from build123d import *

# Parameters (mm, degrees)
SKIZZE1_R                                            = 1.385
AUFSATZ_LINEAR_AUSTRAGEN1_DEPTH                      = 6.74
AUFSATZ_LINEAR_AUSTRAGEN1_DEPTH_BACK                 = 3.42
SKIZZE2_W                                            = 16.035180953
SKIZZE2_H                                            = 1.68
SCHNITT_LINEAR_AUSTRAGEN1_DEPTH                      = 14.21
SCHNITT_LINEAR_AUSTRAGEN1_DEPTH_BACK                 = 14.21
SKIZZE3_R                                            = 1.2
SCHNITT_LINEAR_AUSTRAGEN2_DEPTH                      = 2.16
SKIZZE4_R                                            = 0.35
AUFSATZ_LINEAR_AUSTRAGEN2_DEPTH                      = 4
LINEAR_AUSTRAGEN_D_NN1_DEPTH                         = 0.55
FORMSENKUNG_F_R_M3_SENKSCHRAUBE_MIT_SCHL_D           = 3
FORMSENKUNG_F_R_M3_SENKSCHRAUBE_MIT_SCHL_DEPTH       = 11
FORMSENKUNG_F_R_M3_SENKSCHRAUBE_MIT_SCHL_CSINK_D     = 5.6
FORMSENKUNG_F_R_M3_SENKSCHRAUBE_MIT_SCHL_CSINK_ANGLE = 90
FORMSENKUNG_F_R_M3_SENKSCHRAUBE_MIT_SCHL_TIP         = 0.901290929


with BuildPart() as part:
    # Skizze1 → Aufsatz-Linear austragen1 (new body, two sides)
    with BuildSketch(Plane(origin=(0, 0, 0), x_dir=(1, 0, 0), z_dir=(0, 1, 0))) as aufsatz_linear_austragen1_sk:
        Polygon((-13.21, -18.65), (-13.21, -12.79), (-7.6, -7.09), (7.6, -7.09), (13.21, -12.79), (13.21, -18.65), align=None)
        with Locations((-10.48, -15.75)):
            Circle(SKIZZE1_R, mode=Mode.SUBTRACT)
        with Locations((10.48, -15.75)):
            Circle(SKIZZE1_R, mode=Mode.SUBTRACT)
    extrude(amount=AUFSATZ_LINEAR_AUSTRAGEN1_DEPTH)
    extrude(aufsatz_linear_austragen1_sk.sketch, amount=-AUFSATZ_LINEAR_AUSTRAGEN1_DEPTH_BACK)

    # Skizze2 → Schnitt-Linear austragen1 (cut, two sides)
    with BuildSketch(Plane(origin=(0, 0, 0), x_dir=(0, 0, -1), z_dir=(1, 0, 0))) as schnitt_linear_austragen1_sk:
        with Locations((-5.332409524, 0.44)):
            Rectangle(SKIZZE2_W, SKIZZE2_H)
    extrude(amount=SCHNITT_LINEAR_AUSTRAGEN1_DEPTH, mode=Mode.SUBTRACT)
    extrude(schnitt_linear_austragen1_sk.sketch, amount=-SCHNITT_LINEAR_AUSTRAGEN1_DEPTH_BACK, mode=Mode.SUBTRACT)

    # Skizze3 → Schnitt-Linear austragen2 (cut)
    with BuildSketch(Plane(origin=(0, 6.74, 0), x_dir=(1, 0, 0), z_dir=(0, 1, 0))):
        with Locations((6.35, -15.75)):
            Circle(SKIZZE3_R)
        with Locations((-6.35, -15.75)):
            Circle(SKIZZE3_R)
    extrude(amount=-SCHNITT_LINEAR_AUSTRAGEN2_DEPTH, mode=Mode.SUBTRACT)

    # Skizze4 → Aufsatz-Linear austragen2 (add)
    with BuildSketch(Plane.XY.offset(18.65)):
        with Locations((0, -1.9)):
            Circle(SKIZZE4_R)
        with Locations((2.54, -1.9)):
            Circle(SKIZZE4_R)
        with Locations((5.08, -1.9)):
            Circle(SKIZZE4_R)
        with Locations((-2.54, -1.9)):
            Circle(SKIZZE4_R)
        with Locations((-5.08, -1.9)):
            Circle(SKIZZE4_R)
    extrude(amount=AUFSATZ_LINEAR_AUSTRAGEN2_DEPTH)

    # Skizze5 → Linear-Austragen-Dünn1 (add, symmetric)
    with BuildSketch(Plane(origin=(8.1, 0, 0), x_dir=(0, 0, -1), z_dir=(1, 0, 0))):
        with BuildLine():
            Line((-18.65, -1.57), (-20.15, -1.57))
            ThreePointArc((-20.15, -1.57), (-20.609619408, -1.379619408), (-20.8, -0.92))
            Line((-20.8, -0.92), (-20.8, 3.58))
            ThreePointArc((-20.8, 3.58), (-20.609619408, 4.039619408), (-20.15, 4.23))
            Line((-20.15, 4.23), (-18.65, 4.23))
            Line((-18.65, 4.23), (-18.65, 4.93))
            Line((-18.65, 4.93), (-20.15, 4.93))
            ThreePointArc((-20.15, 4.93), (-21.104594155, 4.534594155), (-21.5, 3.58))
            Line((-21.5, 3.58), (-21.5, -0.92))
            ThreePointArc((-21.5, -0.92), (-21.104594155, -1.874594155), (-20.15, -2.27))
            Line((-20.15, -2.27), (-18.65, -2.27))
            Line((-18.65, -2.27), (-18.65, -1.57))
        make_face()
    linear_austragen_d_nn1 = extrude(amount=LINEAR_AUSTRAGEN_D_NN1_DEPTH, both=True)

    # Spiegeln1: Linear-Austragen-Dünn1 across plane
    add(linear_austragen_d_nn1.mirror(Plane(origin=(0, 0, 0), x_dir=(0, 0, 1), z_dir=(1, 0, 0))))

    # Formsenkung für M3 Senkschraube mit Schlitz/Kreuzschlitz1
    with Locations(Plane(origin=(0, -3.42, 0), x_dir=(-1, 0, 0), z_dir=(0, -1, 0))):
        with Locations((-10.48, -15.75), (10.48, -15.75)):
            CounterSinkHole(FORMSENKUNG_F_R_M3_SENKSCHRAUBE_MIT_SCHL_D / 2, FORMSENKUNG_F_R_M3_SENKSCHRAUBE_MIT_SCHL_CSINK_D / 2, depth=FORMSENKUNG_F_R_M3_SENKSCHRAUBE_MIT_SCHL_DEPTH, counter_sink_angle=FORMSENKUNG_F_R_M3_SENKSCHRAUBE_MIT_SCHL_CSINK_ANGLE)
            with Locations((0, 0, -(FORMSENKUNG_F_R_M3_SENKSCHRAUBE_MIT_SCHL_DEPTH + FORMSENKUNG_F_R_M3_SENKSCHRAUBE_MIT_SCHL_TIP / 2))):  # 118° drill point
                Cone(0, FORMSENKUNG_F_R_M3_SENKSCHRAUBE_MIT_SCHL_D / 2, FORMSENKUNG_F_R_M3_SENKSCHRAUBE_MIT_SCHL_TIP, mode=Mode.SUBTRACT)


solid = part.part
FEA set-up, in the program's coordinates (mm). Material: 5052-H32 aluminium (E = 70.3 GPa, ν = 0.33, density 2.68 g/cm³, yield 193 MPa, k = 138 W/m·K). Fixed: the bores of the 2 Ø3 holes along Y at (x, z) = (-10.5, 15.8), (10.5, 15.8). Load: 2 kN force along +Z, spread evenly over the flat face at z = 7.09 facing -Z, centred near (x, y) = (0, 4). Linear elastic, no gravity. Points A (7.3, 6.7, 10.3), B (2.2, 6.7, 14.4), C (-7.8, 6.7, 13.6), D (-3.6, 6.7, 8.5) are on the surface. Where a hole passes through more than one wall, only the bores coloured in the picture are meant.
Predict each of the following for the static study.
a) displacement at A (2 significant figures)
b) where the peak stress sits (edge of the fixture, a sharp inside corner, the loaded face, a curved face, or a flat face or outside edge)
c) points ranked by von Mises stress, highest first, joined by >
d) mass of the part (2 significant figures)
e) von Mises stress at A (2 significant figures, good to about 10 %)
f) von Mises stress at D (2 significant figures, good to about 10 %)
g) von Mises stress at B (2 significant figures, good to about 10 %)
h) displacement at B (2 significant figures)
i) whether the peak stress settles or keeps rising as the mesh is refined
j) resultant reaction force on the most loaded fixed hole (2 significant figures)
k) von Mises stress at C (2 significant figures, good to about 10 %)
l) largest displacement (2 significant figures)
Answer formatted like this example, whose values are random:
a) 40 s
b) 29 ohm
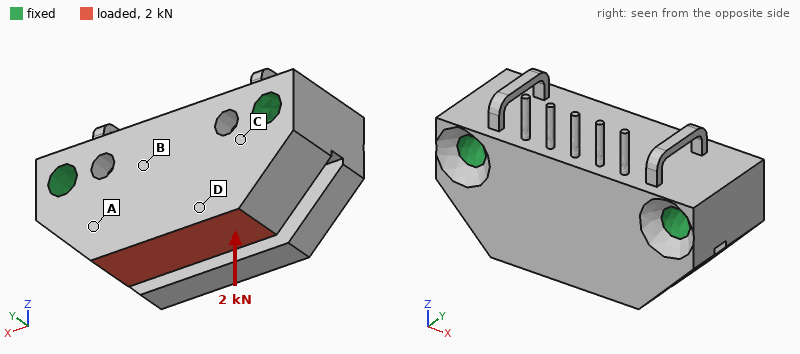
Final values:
a) 4.1 µm
b) edge of the fixture
c) C > A > D > B
d) 6.4 g
e) 34 MPa
f) 23 MPa
g) 15 MPa
h) 6.4 µm
i) keeps rising
j) 1.1 kN
k) 51 MPa
l) 9.1 µm
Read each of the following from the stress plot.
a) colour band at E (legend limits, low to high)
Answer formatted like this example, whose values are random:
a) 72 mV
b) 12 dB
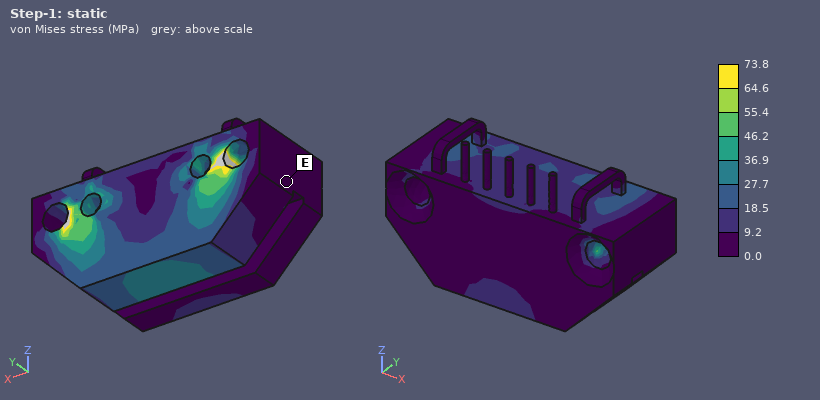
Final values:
a) 0.0 to 9.2 MPa
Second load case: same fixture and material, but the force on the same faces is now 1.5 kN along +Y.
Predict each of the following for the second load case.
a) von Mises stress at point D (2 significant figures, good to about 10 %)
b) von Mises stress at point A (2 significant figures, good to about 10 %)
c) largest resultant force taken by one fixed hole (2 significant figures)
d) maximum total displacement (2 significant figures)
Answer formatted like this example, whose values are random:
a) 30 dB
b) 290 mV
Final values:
a) 41 MPa
b) 73 MPa
c) 750 N
d) 33 µm
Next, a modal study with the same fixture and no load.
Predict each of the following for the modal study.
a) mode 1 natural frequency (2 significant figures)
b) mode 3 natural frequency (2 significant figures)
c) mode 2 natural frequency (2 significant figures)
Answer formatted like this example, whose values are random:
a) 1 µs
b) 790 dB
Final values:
a) 29 kHz
b) 29 kHz
c) 29 kHz
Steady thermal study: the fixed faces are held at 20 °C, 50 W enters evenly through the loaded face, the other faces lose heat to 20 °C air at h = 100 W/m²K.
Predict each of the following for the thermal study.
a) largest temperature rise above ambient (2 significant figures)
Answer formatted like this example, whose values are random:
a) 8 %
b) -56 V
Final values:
a) 38 K
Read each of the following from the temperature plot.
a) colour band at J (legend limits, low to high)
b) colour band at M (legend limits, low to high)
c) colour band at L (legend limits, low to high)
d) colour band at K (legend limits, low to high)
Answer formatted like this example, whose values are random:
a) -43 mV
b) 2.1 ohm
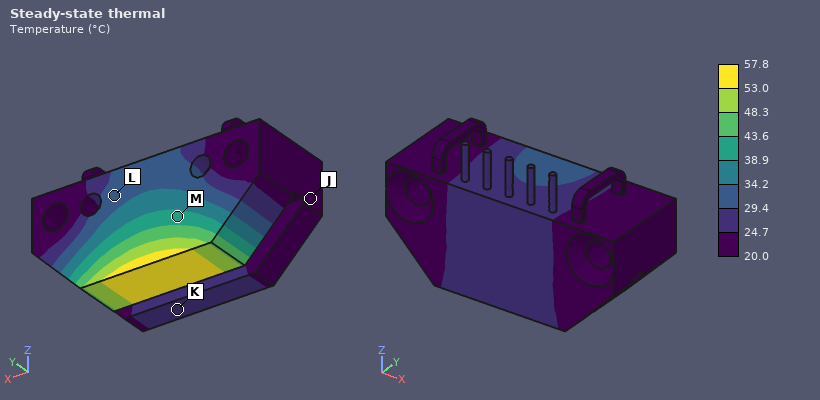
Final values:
a) 20.0 to 24.7 °C
b) 38.9 to 43.6 °C
c) 29.4 to 34.2 °C
d) 24.7 to 29.4 °C
